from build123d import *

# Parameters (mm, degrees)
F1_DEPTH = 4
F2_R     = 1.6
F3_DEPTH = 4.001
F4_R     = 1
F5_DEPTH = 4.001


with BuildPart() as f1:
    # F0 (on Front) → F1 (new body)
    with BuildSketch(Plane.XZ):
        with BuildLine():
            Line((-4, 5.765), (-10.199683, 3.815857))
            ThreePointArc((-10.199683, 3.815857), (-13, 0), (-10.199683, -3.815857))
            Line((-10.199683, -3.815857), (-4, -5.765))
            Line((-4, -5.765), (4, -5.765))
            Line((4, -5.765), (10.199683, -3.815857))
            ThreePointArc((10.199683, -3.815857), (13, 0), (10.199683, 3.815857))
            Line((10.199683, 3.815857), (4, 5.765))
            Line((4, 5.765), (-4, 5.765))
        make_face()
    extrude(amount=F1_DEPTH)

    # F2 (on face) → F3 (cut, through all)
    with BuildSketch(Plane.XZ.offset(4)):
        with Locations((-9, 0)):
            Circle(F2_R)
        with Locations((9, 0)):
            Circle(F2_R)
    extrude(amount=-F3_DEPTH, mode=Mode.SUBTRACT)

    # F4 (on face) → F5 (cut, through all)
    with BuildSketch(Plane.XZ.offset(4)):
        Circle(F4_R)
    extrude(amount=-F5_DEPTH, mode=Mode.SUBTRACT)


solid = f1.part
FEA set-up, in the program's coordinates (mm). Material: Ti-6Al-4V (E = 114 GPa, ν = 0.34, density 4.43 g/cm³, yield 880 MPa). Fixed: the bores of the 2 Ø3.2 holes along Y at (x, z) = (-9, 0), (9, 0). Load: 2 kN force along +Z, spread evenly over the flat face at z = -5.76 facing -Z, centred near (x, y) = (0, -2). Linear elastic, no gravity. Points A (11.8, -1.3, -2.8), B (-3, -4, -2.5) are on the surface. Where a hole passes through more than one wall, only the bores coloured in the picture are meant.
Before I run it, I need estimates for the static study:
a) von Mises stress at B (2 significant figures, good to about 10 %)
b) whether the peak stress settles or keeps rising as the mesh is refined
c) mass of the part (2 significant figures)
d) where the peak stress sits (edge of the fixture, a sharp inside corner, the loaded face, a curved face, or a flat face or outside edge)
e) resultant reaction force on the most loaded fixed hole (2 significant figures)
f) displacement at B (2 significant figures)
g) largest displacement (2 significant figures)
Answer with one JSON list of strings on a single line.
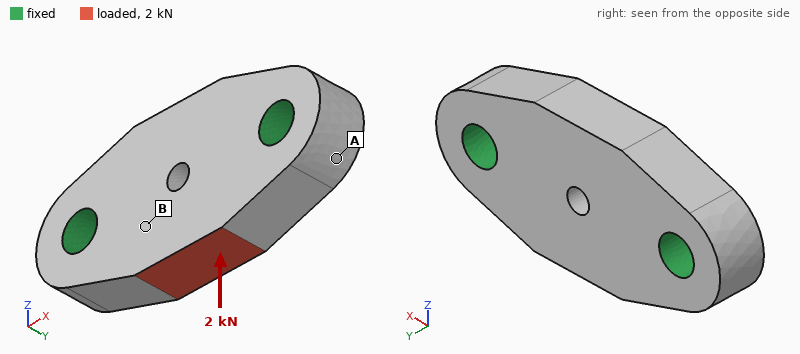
["56 MPa", "keeps rising", "4.0 g", "edge of the fixture", "1.0 kN", "4.9 µm", "7.5 µm"]
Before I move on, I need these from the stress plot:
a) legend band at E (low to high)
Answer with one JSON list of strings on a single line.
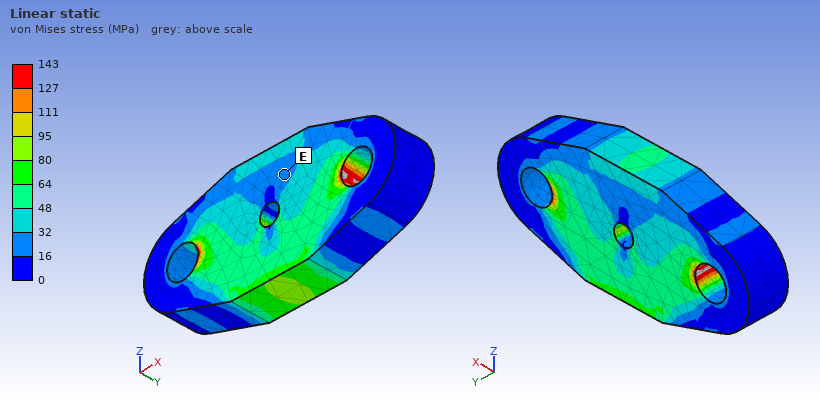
["16 to 32 MPa"]
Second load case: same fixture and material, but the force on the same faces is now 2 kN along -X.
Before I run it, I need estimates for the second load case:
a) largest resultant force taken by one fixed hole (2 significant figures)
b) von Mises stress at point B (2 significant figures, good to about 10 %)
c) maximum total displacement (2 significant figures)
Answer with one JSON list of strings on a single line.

["1.2 kN", "38 MPa", "5.8 µm"]
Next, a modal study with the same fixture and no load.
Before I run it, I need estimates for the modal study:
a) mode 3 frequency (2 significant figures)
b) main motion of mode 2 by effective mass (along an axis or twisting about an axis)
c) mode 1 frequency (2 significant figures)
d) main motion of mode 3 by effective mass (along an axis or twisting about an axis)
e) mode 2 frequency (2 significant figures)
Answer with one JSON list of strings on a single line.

["70 kHz", "twisting about X", "50 kHz", "along Z", "52 kHz"]
